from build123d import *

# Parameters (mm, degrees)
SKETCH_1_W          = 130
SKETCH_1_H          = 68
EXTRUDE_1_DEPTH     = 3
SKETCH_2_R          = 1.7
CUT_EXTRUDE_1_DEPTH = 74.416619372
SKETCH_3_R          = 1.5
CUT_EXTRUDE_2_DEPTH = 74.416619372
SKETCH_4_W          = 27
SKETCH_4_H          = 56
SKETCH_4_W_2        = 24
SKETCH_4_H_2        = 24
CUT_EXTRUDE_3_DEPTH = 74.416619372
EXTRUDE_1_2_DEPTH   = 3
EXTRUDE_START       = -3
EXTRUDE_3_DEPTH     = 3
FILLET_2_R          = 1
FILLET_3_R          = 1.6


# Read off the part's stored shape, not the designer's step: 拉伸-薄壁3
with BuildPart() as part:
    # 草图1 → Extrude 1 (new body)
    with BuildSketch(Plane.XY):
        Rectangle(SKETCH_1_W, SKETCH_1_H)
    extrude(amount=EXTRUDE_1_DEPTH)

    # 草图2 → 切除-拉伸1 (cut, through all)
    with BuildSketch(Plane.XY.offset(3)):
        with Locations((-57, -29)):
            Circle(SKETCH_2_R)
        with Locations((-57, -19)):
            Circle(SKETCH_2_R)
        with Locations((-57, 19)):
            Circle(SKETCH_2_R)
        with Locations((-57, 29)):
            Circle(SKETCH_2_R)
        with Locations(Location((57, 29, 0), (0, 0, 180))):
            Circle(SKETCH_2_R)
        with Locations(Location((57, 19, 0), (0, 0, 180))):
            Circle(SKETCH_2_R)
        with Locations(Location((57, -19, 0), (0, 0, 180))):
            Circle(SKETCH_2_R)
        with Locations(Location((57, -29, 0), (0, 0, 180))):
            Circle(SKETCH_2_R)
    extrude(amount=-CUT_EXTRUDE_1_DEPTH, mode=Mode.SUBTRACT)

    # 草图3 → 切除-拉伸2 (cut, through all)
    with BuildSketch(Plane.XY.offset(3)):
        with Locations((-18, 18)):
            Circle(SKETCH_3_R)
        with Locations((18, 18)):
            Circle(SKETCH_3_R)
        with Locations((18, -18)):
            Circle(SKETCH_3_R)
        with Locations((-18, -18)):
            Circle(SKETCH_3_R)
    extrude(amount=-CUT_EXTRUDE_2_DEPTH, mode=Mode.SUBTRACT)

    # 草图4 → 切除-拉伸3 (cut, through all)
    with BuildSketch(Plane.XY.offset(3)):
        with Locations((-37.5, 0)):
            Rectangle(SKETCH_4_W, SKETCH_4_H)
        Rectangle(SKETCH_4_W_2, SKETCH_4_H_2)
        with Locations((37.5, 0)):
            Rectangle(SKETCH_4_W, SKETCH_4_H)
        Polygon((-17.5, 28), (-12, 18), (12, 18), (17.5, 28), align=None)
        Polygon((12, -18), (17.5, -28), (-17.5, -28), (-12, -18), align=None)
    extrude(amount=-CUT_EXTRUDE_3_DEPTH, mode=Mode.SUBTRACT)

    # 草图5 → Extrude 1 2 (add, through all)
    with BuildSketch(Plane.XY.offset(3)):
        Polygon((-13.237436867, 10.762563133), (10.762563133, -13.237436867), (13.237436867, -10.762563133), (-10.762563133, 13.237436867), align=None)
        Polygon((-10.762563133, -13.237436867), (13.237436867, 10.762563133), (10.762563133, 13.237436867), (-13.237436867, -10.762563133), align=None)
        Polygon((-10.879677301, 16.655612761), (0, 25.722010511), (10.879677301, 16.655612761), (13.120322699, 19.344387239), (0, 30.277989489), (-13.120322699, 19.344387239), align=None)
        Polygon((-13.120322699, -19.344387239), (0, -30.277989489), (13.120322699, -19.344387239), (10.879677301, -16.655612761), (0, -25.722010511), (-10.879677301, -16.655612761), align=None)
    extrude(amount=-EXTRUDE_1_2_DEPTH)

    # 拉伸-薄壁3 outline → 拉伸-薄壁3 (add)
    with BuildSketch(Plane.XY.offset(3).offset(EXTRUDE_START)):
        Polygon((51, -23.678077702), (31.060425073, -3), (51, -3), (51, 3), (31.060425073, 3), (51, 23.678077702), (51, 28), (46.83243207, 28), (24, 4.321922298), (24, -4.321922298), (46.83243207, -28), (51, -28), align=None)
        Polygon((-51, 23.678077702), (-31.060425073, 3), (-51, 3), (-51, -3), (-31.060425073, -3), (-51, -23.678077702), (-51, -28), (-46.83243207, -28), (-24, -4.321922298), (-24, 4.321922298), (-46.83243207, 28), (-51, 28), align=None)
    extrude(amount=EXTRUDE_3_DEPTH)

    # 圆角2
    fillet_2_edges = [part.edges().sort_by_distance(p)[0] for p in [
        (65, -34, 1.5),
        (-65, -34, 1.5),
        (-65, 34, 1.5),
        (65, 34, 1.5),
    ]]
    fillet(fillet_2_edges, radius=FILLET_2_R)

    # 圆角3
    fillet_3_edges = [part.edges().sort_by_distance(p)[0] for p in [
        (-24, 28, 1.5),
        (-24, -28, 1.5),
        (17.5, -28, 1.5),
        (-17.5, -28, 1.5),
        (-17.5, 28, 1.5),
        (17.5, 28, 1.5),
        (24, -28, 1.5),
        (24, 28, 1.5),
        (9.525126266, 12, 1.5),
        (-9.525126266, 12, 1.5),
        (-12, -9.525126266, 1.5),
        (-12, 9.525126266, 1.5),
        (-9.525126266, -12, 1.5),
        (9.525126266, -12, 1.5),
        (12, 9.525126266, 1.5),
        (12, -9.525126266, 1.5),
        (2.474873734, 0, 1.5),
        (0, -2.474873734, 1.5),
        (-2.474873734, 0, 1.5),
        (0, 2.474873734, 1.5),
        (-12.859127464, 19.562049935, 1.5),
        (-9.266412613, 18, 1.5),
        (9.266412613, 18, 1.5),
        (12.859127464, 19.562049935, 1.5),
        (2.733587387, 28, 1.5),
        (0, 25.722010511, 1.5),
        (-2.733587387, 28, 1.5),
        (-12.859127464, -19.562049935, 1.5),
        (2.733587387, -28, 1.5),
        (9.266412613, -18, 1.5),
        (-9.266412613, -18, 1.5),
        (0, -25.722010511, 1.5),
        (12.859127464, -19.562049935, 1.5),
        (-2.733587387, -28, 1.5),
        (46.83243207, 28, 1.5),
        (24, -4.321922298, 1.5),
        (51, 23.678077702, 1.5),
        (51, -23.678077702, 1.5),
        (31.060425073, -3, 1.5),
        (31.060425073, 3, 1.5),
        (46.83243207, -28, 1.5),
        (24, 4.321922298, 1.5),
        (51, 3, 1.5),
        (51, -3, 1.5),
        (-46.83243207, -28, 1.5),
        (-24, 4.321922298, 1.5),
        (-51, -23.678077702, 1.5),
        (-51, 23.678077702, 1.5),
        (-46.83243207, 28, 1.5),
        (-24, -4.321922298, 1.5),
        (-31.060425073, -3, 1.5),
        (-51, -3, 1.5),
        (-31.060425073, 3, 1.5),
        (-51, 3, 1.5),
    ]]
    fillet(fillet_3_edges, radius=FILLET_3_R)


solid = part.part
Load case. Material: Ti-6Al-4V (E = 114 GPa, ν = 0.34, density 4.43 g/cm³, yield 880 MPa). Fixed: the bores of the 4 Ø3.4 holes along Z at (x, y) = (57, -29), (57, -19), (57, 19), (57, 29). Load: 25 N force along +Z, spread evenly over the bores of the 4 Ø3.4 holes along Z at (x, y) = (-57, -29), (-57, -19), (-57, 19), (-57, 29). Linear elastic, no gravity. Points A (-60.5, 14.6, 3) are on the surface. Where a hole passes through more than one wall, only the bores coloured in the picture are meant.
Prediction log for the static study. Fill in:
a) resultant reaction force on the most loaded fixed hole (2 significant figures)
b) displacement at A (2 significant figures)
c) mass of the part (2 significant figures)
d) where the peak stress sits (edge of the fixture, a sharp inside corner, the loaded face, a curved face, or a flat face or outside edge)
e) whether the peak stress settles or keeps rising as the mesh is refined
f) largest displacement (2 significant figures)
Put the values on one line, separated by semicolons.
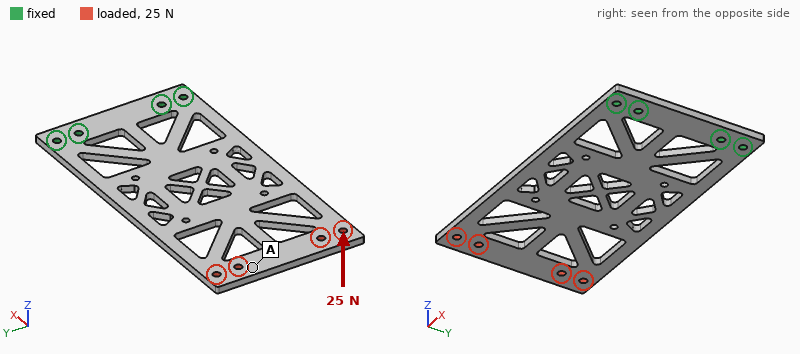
7.7 N; 1.6 mm; 82 g; a sharp inside corner; keeps rising; 1.7 mm
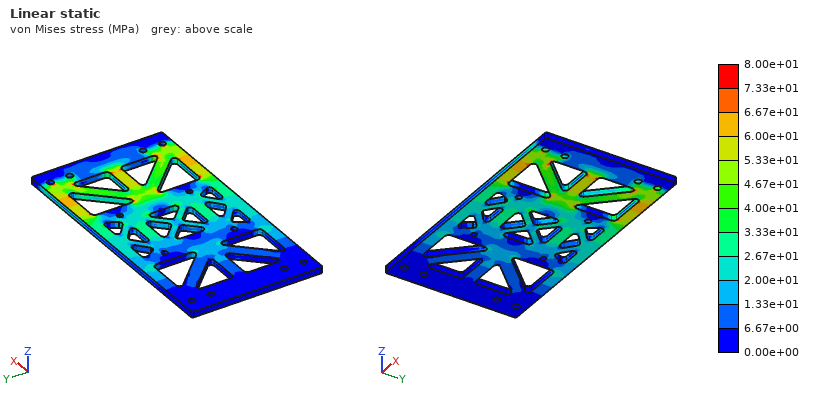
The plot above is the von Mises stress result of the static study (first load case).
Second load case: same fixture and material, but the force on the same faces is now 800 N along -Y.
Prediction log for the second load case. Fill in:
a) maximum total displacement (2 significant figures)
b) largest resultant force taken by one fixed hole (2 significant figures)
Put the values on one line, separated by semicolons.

0.14 mm; 1.6 kN
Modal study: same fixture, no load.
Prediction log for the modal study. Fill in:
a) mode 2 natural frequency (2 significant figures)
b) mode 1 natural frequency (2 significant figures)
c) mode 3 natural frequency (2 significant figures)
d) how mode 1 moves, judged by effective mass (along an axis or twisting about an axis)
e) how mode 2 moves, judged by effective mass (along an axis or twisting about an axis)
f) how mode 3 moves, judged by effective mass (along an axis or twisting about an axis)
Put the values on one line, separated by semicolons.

550 Hz; 130 Hz; 840 Hz; along Z; twisting about X; along Z
